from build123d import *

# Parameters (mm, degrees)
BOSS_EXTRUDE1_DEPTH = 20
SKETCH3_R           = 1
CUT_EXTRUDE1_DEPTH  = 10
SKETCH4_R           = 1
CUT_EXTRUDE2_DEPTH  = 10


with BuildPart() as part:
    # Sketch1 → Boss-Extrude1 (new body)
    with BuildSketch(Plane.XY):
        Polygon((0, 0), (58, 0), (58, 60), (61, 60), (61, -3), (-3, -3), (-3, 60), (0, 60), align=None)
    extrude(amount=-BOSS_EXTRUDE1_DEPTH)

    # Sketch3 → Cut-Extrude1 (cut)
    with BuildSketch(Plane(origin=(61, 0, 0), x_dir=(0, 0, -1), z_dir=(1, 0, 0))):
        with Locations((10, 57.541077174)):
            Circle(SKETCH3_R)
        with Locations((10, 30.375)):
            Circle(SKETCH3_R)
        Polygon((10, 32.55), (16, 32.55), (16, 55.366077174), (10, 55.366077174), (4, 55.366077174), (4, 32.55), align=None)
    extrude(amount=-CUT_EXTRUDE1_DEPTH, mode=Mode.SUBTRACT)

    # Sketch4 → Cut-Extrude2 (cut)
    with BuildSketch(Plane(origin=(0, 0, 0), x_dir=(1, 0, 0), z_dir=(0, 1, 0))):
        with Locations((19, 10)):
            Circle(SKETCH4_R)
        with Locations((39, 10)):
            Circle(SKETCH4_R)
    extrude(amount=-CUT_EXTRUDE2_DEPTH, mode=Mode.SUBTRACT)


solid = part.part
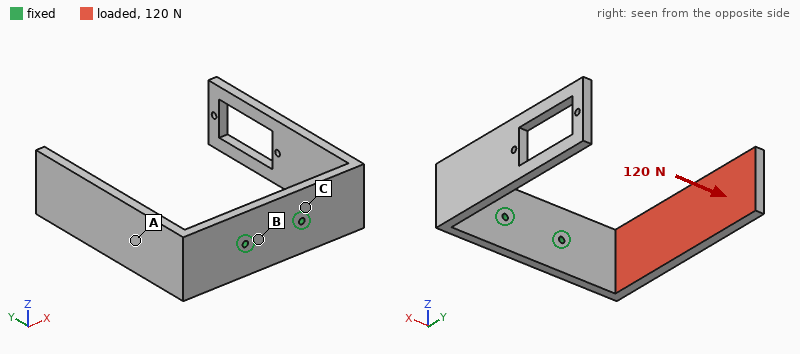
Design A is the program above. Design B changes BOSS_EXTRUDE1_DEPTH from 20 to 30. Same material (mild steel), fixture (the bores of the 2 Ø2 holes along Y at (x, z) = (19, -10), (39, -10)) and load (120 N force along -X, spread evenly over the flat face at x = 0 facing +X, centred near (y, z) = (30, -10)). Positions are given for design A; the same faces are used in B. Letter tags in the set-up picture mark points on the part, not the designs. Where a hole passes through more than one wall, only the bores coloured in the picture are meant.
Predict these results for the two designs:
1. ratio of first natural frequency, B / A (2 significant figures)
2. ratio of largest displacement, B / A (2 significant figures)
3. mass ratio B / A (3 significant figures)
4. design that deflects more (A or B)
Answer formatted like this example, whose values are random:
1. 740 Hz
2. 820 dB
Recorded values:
1. 0.98
2. 0.68
3. 1.54
4. A
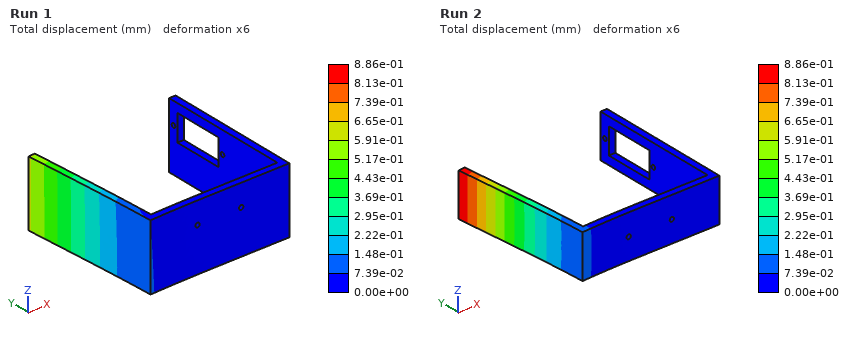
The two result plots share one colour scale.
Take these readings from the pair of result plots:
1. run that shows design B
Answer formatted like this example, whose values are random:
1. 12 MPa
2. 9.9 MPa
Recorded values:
1. Run 1
